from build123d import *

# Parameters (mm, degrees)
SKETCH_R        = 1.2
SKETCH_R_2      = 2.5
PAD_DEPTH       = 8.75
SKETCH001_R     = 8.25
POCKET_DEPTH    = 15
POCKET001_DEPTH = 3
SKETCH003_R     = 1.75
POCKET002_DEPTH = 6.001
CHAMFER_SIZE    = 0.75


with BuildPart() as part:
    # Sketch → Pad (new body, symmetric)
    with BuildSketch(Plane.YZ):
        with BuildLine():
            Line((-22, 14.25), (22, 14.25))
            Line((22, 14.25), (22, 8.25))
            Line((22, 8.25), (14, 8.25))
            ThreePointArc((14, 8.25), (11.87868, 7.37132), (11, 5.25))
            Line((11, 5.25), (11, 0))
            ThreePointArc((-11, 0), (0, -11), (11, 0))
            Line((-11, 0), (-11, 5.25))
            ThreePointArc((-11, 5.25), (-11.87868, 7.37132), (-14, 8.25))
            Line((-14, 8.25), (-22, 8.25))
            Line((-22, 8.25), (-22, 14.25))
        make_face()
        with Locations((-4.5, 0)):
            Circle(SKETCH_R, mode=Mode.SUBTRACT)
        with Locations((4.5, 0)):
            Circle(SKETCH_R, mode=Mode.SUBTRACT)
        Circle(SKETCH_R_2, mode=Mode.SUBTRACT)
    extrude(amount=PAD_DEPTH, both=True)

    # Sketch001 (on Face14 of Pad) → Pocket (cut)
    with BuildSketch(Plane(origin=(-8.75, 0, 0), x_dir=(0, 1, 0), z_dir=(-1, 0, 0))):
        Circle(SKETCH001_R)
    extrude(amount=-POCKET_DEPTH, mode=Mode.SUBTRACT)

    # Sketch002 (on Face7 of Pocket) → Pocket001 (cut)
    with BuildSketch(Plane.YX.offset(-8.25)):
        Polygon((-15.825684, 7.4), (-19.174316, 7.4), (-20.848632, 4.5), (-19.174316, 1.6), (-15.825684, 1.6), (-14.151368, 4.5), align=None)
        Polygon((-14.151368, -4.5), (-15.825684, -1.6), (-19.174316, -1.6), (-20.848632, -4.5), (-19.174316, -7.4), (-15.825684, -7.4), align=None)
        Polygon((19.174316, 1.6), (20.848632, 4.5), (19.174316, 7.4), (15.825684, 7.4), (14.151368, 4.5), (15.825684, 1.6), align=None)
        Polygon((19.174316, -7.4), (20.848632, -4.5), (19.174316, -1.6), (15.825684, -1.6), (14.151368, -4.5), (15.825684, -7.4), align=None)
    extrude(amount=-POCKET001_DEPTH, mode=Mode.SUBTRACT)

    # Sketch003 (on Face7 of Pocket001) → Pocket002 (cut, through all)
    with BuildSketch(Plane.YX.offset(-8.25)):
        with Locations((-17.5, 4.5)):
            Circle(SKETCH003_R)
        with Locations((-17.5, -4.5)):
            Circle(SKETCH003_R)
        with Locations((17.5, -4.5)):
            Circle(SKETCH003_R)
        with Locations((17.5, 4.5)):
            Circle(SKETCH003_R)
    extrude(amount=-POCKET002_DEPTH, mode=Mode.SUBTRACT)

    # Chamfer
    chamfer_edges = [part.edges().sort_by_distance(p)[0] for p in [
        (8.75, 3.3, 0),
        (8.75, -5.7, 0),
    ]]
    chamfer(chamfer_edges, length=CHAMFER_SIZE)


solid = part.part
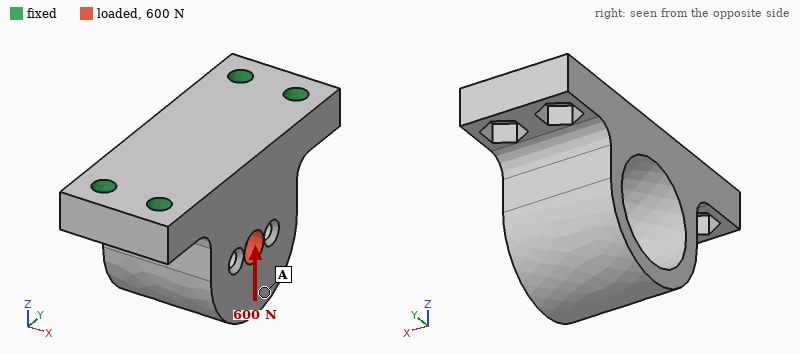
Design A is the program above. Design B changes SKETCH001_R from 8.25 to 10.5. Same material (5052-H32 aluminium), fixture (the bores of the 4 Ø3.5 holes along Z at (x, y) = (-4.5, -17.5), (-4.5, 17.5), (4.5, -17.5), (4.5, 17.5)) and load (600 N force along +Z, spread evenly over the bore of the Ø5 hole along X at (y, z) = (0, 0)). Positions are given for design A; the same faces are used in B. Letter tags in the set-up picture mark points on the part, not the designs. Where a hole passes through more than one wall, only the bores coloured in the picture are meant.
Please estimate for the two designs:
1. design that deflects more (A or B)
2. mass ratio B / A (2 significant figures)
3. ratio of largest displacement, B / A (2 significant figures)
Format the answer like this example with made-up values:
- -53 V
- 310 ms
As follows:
- B
- 0.73
- 1.2
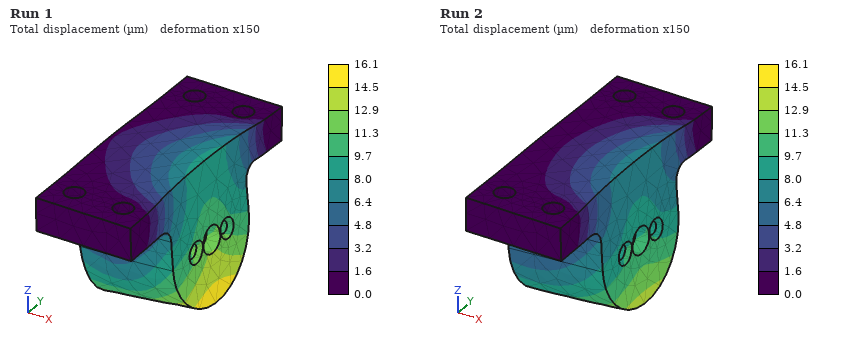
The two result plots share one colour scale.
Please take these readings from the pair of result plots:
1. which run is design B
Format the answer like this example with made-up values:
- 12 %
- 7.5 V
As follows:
- Run 1
